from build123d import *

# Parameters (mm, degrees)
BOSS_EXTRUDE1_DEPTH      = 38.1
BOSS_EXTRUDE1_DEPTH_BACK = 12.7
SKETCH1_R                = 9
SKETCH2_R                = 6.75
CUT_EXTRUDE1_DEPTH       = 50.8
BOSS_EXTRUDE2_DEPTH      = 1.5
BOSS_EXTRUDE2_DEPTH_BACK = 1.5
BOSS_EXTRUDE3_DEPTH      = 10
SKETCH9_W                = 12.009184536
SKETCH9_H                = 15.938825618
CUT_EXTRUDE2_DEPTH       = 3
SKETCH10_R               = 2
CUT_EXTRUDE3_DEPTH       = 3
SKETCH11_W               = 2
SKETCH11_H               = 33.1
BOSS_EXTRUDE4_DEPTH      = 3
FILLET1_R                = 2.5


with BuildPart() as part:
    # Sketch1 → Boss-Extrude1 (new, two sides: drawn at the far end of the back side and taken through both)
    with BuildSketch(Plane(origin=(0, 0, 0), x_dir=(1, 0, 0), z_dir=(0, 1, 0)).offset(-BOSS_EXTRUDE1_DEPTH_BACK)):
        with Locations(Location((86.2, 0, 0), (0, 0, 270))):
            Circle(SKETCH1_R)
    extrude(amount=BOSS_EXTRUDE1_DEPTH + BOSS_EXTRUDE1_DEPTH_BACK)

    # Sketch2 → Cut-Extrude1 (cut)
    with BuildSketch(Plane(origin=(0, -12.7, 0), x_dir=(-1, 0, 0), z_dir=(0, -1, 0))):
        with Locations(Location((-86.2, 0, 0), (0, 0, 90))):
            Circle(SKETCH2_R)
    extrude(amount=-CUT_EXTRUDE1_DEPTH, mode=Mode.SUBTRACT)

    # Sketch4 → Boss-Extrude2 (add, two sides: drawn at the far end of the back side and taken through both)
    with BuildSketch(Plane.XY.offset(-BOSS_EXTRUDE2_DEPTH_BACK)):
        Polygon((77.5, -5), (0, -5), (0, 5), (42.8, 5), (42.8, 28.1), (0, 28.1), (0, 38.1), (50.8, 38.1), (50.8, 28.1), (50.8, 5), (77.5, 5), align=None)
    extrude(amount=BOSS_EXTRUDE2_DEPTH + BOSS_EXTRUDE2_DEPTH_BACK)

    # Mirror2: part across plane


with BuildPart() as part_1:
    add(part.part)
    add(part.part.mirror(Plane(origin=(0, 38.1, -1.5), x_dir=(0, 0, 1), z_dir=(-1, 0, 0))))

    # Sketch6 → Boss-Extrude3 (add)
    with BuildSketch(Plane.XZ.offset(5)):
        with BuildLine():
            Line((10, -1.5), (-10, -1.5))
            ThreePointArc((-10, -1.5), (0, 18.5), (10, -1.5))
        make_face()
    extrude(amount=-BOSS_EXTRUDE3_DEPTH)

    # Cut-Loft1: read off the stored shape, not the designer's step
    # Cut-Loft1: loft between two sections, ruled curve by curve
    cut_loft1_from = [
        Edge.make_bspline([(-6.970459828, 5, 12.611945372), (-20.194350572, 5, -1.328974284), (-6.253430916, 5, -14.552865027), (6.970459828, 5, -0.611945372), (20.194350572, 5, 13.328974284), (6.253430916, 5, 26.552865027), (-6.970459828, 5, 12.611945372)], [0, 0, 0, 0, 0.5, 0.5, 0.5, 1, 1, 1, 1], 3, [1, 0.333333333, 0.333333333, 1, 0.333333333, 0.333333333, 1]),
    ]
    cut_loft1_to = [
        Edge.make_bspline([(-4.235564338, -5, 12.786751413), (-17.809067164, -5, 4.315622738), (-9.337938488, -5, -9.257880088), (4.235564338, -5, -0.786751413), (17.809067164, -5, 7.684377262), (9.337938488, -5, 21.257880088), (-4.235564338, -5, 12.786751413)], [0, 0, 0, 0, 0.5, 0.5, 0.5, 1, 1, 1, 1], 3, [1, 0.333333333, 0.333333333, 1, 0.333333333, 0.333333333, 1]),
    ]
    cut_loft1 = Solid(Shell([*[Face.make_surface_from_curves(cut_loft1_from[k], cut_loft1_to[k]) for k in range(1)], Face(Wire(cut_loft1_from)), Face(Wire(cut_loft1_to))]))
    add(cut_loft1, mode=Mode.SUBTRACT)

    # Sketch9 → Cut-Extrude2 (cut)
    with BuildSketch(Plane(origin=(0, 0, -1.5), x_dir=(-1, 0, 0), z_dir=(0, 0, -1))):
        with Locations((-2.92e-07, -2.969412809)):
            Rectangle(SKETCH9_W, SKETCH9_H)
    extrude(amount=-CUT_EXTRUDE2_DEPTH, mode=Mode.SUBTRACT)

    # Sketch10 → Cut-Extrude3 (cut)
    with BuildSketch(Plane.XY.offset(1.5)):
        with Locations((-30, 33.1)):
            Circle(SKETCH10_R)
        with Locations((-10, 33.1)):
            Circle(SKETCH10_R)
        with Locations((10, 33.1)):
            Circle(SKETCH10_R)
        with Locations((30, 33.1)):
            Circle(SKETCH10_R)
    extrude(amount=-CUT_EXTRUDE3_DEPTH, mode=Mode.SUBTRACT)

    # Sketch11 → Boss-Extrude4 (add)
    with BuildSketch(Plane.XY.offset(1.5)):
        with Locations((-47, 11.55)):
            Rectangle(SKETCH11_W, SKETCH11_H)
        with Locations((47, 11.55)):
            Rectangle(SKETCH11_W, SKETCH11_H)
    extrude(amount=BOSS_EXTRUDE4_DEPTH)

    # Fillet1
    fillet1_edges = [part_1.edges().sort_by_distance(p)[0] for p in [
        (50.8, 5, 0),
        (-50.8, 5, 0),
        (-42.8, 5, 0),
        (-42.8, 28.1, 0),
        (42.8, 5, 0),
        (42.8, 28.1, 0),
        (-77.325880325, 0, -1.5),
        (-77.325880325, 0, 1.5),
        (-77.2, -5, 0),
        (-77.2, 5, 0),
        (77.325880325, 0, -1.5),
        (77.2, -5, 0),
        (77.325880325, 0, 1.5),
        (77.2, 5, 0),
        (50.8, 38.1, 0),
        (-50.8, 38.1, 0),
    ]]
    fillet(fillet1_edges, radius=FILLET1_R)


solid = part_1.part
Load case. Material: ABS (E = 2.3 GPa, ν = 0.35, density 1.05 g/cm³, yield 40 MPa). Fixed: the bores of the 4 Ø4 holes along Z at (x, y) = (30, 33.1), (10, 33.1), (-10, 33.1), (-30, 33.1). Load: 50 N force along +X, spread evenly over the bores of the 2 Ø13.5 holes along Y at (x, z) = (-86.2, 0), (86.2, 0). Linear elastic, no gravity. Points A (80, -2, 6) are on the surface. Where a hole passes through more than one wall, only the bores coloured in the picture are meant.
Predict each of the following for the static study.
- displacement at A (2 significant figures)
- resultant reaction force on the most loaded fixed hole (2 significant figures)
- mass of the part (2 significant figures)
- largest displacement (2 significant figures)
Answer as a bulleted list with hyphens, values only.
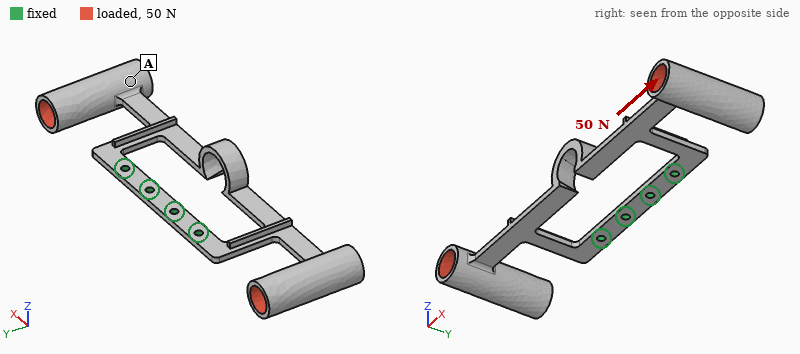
- 0.49 mm
- 26 N
- 23 g
- 0.89 mm
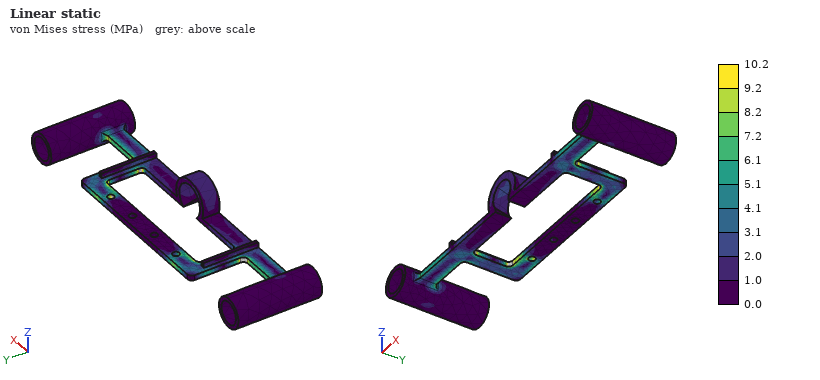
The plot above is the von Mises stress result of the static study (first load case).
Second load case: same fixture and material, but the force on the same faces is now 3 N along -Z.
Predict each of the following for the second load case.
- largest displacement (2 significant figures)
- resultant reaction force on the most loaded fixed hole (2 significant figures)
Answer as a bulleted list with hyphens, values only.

- 2.3 mm
- 1.8 N
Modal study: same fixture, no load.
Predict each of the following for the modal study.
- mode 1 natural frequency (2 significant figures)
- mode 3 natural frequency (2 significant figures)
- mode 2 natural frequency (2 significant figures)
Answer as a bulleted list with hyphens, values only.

- 56 Hz
- 110 Hz
- 57 Hz
